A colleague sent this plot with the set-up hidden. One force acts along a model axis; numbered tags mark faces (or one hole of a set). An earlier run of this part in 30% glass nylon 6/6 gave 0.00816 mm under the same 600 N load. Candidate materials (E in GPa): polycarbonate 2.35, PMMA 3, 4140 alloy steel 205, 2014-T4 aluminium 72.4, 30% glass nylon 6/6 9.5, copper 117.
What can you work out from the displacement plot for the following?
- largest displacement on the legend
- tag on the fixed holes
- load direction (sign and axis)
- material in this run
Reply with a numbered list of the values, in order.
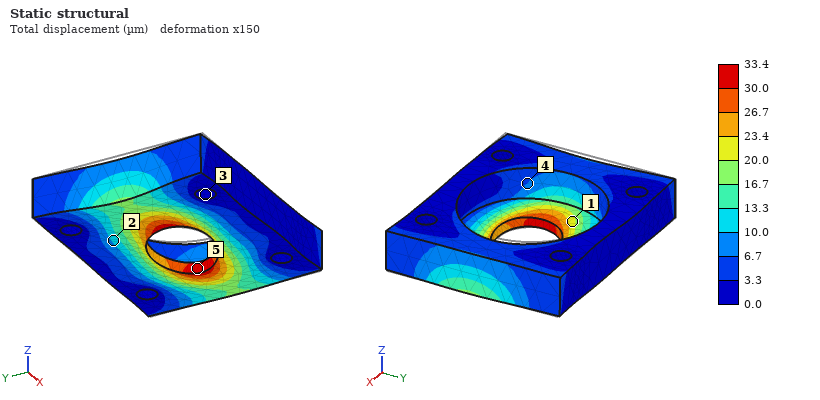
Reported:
1. 33.4 µm
2. 3
3. +X
4. polycarbonate
